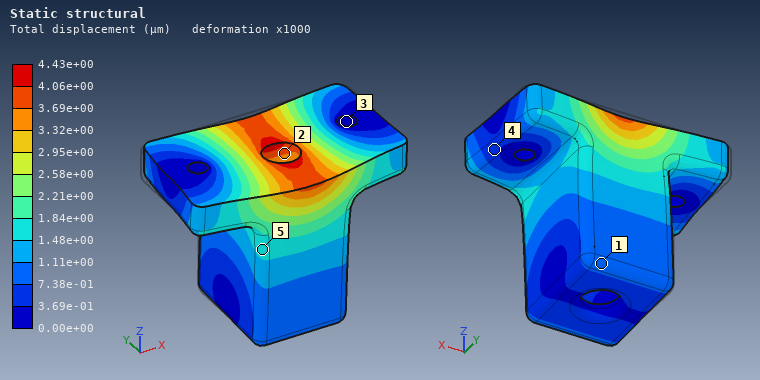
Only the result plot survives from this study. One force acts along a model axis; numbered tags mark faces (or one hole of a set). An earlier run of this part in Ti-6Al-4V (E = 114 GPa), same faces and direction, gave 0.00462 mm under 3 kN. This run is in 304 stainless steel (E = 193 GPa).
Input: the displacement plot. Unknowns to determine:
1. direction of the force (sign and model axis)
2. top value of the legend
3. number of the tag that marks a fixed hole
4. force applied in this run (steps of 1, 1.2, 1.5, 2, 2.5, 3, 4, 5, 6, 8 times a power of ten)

-Y
4.43e+00 µm
3
5 kN
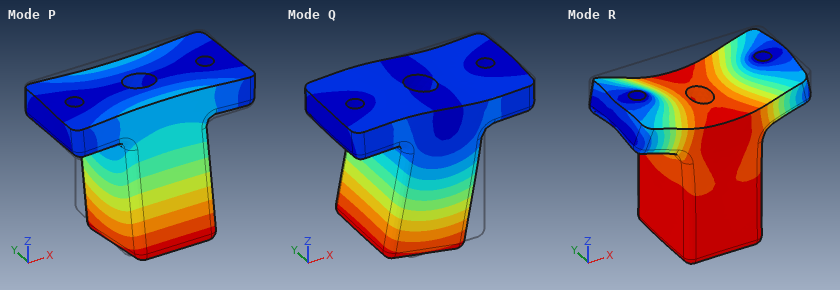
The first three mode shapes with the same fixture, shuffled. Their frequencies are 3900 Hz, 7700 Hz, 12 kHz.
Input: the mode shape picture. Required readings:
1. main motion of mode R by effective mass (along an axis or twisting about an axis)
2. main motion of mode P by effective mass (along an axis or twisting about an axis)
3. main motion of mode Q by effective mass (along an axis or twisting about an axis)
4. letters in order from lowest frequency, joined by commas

along Z
along Y
along X
P, Q, R
